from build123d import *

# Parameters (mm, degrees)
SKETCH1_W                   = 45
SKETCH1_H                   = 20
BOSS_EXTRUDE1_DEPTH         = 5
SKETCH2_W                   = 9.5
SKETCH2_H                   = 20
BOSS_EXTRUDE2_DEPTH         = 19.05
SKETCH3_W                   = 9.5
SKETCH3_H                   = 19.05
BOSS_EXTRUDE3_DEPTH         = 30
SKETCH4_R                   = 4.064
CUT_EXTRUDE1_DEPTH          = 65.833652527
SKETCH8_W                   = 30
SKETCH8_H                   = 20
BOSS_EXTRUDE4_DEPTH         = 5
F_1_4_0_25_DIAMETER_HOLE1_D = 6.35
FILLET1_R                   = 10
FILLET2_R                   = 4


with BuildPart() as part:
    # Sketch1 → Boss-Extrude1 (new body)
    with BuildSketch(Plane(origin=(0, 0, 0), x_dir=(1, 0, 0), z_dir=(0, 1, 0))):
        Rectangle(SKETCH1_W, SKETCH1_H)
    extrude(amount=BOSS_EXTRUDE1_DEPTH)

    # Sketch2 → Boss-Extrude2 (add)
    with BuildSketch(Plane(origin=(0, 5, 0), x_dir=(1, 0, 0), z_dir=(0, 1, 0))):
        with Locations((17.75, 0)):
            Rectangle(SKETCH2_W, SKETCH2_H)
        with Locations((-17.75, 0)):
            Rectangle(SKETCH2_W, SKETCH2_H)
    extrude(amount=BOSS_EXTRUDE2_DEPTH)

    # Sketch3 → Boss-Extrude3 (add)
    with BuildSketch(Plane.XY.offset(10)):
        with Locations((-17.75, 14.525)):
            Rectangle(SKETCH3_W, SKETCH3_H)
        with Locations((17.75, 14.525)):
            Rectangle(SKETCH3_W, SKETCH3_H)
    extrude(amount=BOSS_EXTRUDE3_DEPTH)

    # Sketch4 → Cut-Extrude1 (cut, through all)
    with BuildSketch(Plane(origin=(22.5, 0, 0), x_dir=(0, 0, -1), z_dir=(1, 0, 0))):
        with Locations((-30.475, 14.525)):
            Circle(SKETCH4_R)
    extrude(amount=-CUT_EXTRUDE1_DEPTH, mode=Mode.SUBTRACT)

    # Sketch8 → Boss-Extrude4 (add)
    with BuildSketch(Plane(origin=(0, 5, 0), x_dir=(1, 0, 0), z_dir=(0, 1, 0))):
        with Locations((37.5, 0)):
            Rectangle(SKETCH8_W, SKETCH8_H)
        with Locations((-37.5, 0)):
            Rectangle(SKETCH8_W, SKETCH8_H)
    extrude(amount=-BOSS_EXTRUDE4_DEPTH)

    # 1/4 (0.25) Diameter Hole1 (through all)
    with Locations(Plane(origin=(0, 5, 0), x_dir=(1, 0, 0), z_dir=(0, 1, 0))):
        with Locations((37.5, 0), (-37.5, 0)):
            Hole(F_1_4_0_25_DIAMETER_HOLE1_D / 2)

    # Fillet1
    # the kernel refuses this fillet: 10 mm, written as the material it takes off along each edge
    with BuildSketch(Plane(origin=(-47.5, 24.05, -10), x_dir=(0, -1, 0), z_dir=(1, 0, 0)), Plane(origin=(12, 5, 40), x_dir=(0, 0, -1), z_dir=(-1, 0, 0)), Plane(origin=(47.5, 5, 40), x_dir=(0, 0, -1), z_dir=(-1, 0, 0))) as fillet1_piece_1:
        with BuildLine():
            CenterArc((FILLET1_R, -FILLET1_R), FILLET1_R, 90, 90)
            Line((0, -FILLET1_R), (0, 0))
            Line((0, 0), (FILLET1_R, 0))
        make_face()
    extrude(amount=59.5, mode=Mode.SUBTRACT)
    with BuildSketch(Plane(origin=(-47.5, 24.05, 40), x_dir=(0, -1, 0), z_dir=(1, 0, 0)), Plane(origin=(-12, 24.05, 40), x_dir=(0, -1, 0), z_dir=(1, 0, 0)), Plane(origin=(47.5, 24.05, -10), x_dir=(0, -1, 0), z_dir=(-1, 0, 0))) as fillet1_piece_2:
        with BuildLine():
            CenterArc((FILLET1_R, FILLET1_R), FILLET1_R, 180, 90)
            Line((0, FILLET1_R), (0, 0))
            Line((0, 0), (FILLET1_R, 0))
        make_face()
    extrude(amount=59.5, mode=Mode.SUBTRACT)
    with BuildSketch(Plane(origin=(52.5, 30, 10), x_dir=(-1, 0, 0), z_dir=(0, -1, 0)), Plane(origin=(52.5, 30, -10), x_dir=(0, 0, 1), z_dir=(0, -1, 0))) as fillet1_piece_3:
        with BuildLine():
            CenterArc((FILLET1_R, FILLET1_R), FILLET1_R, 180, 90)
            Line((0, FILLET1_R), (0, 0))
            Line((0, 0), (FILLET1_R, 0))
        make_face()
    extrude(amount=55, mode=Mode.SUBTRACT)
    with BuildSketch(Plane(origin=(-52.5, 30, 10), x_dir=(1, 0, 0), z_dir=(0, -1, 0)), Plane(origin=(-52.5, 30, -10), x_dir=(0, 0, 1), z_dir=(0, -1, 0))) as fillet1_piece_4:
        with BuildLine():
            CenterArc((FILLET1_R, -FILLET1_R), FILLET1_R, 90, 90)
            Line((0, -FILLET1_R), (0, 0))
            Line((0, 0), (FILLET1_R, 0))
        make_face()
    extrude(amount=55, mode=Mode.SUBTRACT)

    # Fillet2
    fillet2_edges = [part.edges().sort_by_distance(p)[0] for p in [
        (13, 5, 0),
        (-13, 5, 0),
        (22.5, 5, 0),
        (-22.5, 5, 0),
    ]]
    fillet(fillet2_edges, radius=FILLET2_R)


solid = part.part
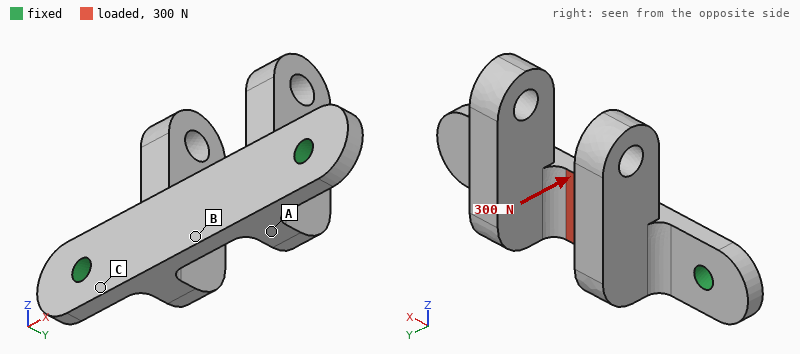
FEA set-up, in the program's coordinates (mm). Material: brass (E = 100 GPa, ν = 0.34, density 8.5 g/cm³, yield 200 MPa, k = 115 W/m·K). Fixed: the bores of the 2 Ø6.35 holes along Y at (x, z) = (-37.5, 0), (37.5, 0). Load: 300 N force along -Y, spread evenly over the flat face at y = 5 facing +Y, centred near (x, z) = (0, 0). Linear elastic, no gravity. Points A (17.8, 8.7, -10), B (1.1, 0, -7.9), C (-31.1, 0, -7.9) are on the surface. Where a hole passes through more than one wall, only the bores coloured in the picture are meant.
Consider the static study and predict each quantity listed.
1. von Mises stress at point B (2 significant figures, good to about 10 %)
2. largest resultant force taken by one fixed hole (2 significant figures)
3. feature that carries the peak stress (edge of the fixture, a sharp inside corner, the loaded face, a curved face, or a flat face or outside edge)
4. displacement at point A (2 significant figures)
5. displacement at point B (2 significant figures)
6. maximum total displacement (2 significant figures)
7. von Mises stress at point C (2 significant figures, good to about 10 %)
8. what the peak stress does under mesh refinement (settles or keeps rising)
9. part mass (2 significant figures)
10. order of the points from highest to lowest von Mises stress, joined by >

25 MPa
150 N
edge of the fixture
15 µm
27 µm
29 µm
18 MPa
keeps rising
220 g
B > C > A
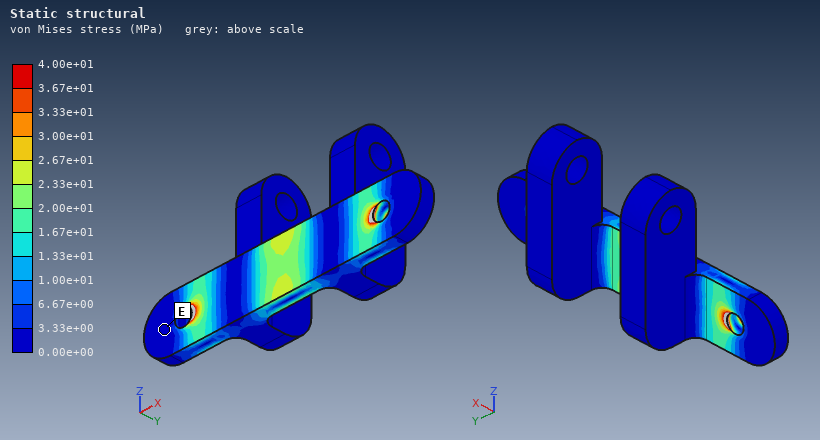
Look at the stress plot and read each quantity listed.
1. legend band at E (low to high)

0.00e+00 to 3.33e+00 MPa
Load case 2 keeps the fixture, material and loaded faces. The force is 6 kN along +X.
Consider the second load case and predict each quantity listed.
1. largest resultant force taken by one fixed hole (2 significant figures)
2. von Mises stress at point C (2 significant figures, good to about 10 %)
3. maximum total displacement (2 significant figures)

3.0 kN
25 MPa
13 µm
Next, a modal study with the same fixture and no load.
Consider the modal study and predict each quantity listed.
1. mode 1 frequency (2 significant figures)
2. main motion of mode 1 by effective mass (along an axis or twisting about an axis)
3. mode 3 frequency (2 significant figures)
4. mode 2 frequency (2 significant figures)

1200 Hz
along Y
1800 Hz
1800 Hz
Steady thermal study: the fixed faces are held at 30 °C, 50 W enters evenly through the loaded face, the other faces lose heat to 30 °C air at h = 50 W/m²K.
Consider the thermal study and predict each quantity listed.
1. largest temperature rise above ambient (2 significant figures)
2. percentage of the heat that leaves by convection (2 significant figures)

54 K
23 %
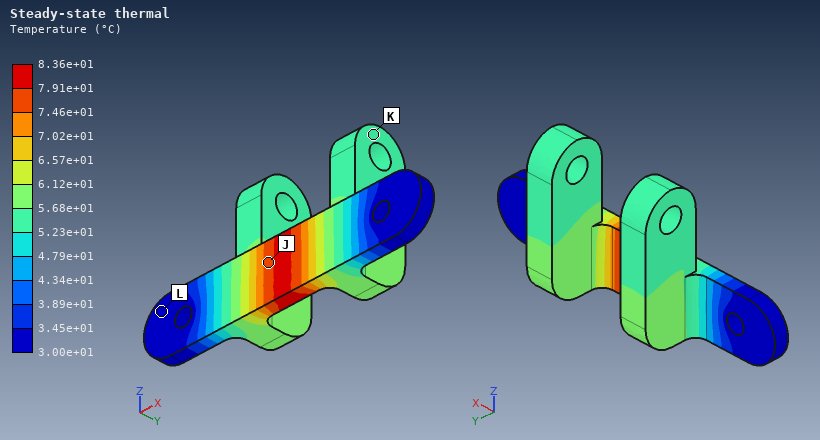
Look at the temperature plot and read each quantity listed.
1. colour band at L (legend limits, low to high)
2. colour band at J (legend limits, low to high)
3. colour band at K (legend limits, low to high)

3.00e+01 to 3.45e+01 °C
7.46e+01 to 7.91e+01 °C
5.23e+01 to 5.68e+01 °C
